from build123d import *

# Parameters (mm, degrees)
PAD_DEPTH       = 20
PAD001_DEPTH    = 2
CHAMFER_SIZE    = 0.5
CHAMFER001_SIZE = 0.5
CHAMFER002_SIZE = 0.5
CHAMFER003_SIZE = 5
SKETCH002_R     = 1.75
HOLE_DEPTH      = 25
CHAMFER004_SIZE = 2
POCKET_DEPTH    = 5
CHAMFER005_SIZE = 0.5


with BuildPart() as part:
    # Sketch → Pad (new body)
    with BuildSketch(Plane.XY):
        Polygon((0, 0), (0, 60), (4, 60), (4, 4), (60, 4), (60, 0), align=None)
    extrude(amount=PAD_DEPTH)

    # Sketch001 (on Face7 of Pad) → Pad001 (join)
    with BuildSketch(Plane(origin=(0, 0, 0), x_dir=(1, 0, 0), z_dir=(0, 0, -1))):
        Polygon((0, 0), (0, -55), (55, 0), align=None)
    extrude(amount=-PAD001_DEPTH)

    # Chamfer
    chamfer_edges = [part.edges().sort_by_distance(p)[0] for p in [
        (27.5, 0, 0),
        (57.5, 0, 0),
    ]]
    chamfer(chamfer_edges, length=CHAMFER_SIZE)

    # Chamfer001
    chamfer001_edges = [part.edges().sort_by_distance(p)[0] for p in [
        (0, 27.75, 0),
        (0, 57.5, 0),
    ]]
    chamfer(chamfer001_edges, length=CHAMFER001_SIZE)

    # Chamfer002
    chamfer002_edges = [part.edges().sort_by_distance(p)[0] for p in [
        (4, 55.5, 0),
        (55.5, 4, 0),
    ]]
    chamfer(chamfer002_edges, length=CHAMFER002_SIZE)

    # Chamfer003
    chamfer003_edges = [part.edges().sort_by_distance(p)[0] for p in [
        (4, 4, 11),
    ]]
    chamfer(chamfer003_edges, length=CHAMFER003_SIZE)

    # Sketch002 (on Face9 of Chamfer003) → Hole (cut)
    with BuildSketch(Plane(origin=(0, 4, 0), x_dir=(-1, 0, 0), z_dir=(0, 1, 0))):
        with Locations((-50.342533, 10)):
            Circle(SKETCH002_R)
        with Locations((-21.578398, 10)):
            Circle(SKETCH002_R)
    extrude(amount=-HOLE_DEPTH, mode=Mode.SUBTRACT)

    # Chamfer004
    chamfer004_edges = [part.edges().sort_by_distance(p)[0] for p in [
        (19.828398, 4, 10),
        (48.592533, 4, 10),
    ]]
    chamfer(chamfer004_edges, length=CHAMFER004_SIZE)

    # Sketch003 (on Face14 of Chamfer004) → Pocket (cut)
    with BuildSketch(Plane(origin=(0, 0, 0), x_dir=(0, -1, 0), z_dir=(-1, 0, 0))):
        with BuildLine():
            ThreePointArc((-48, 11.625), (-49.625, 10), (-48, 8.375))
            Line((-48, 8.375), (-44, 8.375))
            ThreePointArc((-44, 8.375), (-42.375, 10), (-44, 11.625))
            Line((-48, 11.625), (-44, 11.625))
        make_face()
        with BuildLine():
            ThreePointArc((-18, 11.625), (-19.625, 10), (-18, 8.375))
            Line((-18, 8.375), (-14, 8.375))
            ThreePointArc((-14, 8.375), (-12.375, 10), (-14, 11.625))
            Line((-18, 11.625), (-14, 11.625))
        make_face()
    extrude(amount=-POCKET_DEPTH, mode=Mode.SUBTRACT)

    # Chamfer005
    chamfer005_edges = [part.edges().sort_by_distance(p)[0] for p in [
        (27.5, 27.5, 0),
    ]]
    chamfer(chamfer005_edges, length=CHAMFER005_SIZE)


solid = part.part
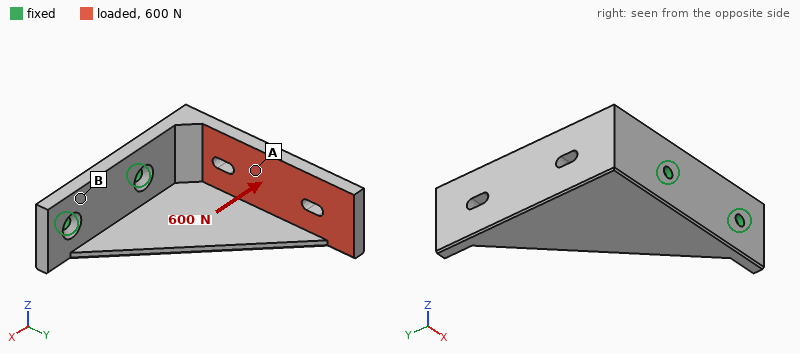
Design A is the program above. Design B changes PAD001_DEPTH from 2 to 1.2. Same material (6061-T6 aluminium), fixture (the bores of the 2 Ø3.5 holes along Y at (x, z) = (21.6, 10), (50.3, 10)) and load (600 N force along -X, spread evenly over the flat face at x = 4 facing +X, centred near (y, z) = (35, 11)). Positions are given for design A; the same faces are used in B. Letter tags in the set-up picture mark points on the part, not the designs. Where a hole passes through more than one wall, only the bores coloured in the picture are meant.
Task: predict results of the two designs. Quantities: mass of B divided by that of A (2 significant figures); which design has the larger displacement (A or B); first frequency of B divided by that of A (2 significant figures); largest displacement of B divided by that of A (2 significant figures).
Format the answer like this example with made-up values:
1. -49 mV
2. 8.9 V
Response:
1. 0.92
2. B
3. 0.99
4. 1.2
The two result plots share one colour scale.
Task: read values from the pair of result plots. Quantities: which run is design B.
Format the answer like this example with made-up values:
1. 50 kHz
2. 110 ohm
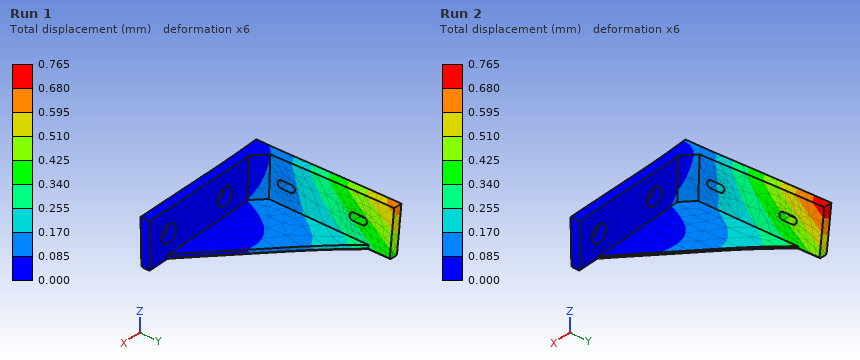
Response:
1. Run 2
